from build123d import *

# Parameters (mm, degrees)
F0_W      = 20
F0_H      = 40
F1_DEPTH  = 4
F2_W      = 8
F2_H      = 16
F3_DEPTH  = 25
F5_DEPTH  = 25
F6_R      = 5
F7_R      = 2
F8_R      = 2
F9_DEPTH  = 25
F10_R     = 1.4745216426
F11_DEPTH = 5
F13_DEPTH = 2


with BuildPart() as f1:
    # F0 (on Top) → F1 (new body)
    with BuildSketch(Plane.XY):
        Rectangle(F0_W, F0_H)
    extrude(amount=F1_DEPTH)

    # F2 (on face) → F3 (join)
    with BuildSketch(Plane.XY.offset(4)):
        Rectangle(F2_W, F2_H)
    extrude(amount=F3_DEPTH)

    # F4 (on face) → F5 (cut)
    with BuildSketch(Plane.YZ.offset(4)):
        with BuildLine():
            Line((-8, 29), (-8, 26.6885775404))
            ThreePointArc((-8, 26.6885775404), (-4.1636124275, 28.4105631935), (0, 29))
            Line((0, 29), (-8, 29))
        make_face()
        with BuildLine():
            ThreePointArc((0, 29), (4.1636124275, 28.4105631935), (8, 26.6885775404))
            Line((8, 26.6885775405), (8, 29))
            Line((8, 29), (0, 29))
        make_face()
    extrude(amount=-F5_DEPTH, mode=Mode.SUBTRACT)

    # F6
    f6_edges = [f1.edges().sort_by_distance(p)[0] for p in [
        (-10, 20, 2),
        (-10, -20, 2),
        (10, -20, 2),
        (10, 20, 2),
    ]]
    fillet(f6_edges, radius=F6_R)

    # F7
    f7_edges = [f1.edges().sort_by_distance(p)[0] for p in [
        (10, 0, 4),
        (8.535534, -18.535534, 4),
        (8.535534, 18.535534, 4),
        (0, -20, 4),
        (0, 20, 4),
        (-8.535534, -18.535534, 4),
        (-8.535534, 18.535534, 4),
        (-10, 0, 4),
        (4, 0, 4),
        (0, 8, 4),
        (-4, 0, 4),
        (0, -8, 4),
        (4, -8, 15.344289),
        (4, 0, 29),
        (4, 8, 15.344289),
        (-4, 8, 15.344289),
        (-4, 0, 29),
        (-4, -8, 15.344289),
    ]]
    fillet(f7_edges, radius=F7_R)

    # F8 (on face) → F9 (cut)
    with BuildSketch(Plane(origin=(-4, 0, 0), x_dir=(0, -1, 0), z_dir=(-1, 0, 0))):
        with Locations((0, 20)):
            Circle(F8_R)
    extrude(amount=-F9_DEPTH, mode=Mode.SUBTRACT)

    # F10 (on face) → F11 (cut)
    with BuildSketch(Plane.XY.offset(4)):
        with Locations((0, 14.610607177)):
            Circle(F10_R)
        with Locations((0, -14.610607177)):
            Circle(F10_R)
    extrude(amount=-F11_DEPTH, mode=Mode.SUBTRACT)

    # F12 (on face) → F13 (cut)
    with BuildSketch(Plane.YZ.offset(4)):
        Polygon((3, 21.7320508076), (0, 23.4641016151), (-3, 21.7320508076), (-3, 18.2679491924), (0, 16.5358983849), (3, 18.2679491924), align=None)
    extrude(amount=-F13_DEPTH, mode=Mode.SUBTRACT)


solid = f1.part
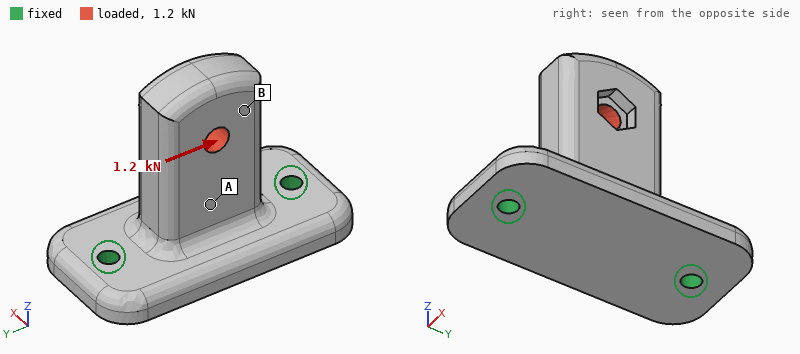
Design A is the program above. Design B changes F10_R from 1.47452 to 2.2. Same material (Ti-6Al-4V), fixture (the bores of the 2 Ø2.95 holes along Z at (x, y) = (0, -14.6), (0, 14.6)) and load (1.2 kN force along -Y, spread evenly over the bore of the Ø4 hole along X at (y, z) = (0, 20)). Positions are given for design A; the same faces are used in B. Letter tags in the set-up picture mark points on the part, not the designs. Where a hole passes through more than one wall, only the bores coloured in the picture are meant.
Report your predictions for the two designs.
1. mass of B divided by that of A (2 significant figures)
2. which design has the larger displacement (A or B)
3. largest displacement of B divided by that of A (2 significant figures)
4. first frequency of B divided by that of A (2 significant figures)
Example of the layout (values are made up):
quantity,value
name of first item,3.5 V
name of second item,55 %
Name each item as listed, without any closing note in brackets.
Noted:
quantity,value
mass of B divided by that of A,0.99
which design has the larger displacement,A
largest displacement of B divided by that of A,0.90
first frequency of B divided by that of A,1.1
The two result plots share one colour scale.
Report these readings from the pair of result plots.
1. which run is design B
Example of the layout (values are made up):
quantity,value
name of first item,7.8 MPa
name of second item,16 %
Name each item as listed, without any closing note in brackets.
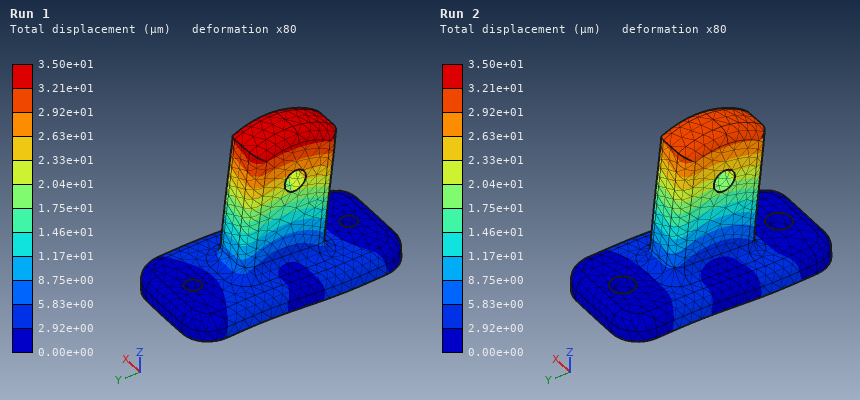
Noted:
quantity,value
which run is design B,Run 2
